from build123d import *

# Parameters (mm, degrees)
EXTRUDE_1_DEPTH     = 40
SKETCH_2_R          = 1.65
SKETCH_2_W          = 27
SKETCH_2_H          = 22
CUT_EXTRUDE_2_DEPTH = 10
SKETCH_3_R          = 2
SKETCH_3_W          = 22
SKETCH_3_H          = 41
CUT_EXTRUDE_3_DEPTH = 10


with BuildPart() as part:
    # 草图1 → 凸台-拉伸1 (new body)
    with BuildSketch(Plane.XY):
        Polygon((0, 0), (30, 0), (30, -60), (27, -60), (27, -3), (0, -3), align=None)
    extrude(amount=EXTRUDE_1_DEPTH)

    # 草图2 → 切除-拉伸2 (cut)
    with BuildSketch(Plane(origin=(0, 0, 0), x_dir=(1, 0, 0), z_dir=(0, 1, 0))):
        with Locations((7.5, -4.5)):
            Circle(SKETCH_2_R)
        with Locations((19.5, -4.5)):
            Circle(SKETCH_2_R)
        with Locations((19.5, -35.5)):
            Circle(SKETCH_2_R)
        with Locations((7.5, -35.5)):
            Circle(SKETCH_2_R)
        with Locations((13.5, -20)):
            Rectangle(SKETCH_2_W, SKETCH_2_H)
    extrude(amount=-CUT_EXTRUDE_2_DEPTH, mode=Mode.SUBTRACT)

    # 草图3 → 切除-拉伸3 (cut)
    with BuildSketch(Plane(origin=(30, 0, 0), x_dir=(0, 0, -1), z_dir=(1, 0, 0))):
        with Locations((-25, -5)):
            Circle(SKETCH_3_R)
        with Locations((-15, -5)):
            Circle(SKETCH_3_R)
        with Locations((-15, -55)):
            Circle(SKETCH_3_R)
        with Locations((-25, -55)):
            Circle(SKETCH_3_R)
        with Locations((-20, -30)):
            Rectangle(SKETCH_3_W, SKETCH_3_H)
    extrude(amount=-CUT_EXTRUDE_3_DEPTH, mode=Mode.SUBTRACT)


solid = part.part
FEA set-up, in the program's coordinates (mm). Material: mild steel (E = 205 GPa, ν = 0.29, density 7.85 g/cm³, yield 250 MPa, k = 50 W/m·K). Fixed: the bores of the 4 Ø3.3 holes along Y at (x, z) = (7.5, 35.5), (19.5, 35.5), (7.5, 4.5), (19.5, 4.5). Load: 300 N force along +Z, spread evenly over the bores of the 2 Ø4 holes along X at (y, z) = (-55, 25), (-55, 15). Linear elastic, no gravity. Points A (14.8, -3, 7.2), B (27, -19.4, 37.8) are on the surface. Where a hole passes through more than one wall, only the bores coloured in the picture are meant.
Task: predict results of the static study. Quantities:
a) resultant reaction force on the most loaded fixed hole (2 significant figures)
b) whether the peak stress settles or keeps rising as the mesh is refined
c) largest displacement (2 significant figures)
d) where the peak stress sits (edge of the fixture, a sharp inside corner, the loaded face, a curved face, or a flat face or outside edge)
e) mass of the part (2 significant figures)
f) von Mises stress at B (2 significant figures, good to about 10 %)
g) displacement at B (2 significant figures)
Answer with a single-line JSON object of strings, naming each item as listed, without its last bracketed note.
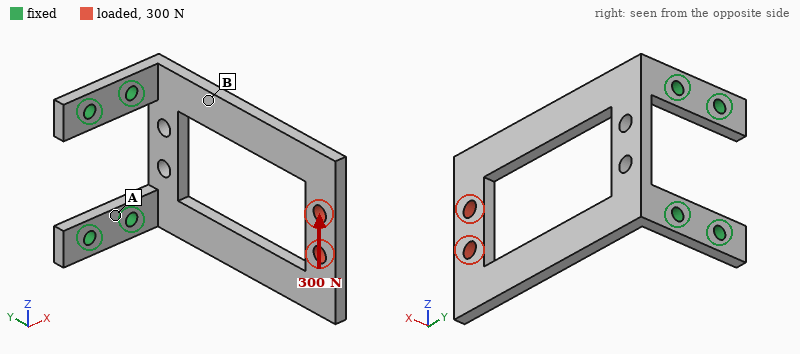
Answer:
{"resultant reaction force on the most loaded fixed hole": "510 N", "whether the peak stress settles or keeps rising as the mesh is refined": "keeps rising", "largest displacement": "0.13 mm", "where the peak stress sits": "edge of the fixture", "mass of the part": "45 g", "von Mises stress at B": "51 MPa", "displacement at B": "0.046 mm"}
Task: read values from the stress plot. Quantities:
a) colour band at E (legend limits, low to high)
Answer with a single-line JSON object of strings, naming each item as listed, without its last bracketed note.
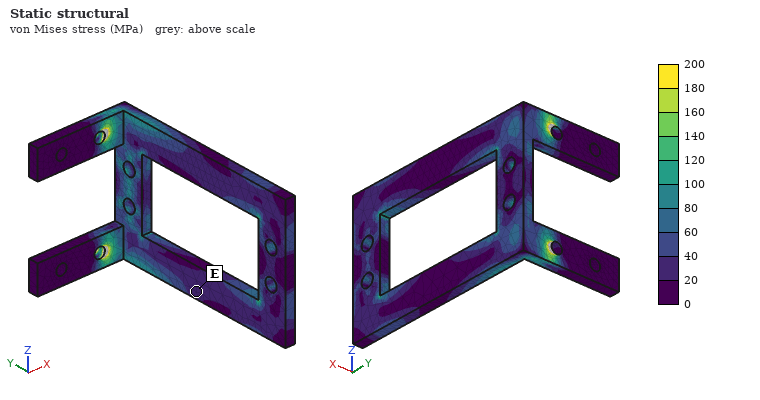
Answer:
{"colour band at E": "20 to 40 MPa"}
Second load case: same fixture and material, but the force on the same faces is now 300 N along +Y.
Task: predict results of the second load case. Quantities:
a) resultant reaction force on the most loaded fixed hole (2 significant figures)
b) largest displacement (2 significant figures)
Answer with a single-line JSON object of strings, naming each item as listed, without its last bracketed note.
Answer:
{"resultant reaction force on the most loaded fixed hole": "160 N", "largest displacement": "72 µm"}
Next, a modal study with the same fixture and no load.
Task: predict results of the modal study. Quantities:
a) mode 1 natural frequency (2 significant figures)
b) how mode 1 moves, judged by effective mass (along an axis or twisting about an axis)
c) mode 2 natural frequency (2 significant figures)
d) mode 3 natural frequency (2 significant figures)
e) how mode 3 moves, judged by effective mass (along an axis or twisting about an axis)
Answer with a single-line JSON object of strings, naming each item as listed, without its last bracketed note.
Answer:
{"mode 1 natural frequency": "490 Hz", "how mode 1 moves, judged by effective mass": "along X", "mode 2 natural frequency": "1600 Hz", "mode 3 natural frequency": "2200 Hz", "how mode 3 moves, judged by effective mass": "along Z"}
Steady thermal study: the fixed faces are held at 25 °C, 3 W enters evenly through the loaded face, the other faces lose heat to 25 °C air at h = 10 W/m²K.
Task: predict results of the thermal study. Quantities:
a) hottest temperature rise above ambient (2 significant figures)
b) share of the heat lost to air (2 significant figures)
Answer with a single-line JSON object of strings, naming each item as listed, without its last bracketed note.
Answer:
{"hottest temperature rise above ambient": "57 K", "share of the heat lost to air": "36 %"}
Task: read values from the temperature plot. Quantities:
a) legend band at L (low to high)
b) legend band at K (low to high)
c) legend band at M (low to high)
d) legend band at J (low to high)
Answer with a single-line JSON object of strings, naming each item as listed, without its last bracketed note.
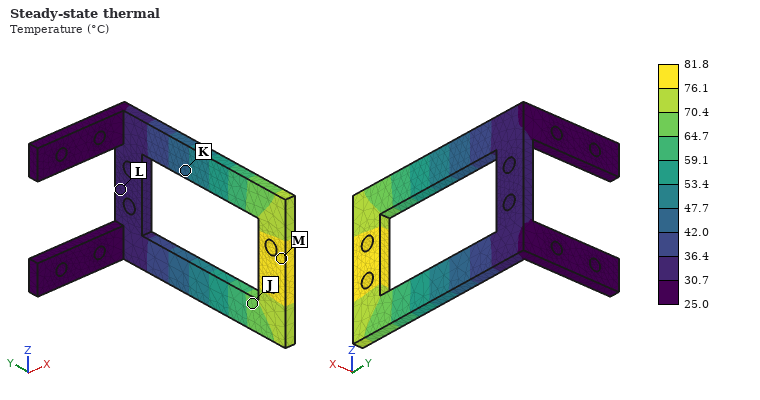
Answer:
{"legend band at L": "30.7 to 36.4 °C", "legend band at K": "42.0 to 47.7 °C", "legend band at M": "76.1 to 81.8 °C", "legend band at J": "64.7 to 70.4 °C"}
